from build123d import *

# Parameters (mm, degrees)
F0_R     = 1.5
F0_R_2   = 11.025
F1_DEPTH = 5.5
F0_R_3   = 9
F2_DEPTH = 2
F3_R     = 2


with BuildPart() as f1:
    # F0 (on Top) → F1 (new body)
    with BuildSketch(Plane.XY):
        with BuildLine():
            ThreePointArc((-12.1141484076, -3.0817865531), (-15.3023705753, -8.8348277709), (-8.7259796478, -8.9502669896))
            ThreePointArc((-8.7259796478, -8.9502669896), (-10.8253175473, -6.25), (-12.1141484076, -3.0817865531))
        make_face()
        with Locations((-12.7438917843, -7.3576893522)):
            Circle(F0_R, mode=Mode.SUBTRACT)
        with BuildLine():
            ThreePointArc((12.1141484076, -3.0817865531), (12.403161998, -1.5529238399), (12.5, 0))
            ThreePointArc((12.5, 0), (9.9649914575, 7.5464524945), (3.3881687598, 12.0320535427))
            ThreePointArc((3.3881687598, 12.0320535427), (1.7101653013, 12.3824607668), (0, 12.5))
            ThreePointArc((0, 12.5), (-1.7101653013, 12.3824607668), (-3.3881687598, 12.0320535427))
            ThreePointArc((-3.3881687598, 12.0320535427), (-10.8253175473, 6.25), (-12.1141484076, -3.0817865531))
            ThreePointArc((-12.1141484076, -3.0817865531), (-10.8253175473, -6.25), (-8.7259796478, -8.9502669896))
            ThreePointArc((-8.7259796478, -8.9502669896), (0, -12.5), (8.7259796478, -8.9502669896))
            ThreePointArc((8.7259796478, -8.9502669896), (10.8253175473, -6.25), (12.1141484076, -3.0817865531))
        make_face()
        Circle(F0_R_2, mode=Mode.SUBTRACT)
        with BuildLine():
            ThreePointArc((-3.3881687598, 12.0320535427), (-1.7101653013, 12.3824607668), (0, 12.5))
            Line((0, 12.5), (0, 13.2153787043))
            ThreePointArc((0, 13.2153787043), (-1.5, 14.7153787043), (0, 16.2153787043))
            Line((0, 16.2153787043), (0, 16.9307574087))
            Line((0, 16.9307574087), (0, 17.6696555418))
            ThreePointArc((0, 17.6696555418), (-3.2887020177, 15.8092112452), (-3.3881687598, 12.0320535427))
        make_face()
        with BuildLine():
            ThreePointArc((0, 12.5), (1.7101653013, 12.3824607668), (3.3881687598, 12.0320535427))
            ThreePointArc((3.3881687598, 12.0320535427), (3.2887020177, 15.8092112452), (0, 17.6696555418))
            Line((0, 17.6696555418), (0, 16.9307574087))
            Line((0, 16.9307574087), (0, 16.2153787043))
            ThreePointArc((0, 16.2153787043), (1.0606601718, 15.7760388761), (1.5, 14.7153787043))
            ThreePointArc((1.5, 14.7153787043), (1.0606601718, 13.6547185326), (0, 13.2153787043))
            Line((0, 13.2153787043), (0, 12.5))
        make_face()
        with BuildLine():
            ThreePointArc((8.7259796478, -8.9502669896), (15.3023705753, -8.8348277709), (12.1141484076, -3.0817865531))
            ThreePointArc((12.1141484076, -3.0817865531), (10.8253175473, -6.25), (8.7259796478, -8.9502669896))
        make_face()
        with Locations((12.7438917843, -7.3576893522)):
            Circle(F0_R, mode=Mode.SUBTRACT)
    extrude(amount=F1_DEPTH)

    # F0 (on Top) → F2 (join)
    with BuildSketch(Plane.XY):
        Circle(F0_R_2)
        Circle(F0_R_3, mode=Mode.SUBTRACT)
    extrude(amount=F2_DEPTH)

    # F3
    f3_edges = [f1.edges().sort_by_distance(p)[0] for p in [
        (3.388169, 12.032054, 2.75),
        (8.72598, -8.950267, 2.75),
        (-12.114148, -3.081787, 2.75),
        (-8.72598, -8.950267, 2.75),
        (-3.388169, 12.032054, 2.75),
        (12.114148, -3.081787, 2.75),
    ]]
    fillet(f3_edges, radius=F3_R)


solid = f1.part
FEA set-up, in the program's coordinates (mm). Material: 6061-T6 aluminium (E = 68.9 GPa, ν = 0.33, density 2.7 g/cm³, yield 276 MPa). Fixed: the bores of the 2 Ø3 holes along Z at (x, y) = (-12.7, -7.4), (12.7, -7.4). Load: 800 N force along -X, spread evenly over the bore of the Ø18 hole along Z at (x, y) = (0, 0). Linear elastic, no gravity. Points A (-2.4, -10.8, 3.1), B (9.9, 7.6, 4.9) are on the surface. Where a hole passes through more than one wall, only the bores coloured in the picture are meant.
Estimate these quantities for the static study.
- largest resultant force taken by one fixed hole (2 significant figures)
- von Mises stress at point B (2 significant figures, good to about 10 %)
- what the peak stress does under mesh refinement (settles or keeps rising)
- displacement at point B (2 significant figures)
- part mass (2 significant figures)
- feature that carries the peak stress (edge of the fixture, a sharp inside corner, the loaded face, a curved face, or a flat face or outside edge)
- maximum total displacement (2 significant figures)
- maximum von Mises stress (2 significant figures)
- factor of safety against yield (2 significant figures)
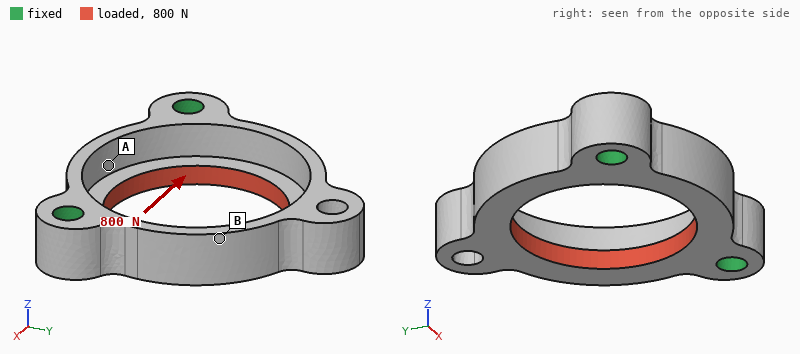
410 N
31 MPa
settles
56 µm
3.6 g
a curved face
61 µm
200 MPa
1.4
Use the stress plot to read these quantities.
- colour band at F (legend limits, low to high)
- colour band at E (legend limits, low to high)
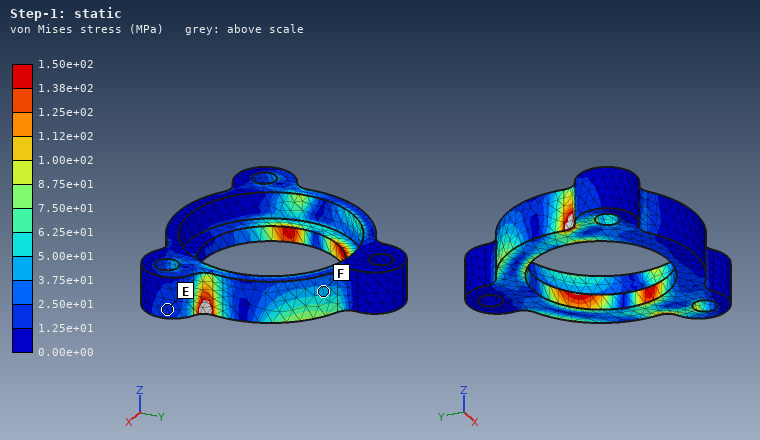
3.75e+01 to 5.00e+01 MPa
1.25e+01 to 2.50e+01 MPa
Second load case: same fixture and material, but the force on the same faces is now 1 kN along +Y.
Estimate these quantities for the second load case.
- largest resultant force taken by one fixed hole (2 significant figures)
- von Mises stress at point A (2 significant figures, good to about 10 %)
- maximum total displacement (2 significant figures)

500 N
11 MPa
41 µm
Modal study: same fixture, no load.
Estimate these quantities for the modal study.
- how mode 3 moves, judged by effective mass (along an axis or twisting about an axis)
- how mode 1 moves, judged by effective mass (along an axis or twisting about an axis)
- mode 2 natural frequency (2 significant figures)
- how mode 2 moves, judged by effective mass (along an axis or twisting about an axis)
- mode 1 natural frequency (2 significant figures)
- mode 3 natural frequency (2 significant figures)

along Y
along Z
11 kHz
along X
5800 Hz
22 kHz
